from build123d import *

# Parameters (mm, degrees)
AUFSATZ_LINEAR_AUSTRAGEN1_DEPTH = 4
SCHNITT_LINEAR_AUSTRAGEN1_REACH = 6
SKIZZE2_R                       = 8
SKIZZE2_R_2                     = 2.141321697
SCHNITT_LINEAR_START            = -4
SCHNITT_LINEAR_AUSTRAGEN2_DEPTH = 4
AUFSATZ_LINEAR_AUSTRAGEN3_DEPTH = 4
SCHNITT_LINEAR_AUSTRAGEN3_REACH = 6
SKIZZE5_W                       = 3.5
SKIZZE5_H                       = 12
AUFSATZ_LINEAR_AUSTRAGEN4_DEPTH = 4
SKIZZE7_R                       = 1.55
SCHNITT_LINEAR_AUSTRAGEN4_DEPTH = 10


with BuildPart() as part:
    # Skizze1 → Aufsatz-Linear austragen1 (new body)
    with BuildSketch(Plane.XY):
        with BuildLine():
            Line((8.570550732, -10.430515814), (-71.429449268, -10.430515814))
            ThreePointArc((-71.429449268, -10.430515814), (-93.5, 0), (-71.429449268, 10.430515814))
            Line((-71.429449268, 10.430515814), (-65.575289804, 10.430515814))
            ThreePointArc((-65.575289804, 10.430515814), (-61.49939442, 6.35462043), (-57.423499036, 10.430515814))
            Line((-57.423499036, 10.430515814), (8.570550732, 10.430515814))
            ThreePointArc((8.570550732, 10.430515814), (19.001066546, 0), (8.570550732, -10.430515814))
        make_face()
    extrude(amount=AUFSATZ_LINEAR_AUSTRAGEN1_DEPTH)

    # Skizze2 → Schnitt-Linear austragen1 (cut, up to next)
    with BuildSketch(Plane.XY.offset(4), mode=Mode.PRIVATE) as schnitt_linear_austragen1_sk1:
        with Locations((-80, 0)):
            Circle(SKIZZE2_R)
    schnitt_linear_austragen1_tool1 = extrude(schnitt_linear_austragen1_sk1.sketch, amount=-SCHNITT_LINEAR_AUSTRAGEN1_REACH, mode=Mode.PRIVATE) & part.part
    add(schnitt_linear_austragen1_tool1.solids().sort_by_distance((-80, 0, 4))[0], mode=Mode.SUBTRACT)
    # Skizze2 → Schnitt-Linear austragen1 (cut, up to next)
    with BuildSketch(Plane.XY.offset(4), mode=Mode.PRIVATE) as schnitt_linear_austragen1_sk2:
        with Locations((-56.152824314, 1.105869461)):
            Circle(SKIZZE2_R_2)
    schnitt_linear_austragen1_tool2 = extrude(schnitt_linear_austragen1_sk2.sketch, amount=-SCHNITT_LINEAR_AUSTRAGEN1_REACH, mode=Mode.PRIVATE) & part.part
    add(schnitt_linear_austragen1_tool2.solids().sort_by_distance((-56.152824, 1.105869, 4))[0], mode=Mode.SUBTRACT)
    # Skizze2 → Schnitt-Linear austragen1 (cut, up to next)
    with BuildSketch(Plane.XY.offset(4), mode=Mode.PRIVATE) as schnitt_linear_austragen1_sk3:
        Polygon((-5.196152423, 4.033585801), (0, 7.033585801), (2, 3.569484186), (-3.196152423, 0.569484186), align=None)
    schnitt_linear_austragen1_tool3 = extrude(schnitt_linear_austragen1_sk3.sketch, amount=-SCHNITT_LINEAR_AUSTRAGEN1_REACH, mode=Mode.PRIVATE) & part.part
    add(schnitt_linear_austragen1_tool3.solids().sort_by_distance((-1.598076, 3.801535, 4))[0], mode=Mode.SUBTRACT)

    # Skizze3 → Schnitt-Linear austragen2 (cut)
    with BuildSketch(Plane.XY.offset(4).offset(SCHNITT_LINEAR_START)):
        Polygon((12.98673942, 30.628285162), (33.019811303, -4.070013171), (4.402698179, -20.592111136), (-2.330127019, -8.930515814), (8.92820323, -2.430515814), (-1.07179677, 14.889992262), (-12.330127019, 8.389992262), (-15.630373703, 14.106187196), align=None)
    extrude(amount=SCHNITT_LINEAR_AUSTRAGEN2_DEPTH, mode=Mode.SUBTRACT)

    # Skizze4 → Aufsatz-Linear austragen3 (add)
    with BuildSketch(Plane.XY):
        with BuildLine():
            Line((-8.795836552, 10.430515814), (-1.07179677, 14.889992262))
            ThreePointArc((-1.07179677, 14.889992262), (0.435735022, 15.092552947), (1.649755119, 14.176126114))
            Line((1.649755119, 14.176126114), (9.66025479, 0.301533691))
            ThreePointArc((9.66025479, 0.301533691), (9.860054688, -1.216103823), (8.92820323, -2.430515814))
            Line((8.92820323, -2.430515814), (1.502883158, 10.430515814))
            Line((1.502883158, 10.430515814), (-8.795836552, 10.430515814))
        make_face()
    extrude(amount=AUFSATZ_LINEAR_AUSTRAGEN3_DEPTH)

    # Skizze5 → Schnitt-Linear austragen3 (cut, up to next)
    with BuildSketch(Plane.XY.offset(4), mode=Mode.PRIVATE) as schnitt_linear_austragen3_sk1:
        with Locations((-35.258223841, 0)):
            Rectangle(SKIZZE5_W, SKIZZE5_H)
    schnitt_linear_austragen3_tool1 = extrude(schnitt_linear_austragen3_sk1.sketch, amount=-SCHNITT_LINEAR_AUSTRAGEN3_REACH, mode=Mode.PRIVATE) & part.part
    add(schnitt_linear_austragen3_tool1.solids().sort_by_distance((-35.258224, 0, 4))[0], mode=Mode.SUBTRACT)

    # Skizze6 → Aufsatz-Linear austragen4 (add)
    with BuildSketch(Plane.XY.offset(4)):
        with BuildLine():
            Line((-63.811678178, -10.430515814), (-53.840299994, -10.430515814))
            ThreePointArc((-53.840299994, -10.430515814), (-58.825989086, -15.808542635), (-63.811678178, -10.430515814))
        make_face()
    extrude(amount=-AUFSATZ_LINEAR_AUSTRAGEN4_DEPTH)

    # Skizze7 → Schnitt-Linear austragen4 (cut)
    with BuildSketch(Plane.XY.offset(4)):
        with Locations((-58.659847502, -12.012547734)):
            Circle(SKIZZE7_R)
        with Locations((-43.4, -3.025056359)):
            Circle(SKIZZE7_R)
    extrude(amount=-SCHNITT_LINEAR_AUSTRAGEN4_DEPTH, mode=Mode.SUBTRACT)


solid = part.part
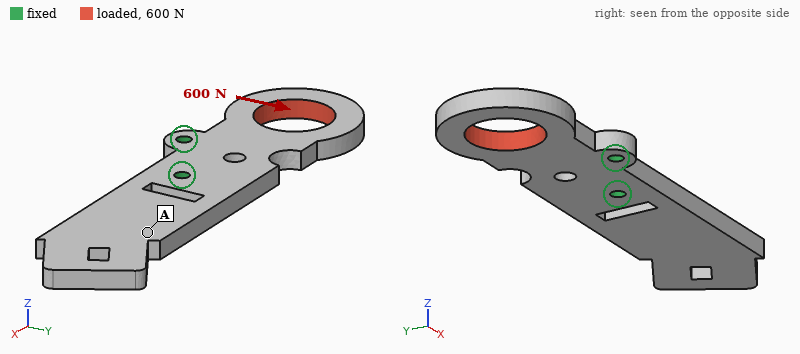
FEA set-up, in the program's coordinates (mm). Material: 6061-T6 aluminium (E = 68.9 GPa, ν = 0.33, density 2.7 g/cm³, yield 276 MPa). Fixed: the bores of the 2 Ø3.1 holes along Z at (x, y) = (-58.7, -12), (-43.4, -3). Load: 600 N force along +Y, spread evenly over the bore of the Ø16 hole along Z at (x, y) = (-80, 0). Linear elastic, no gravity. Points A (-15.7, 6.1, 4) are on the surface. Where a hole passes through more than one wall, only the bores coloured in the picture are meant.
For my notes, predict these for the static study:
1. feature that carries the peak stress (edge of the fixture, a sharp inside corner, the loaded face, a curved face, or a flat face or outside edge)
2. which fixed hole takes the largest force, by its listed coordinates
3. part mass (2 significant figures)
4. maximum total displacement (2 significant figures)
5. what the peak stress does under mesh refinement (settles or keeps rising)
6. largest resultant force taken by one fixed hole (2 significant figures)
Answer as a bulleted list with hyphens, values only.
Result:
- a sharp inside corner
- (-58.7, -12)
- 20 g
- 85 µm
- keeps rising
- 1.2 kN
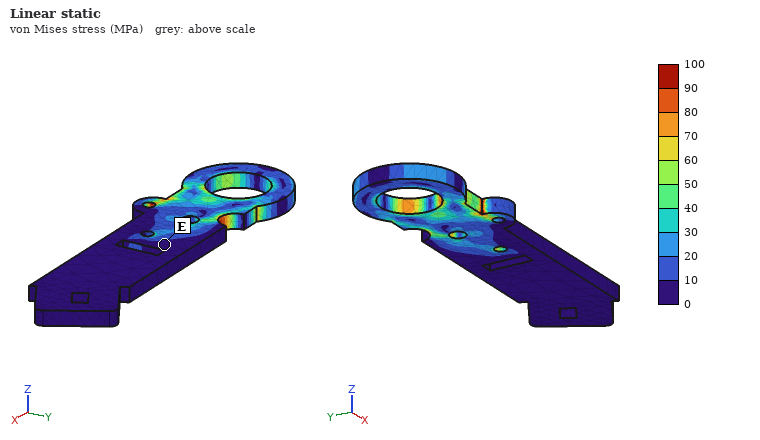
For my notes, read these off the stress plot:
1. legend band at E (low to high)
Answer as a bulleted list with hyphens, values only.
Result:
- 0 to 10 MPa
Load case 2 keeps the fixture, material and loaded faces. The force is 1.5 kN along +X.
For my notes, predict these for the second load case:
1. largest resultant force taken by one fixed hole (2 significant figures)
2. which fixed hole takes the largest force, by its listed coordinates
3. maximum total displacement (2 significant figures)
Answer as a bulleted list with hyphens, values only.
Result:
- 1.2 kN
- (-43.4, -3)
- 44 µm
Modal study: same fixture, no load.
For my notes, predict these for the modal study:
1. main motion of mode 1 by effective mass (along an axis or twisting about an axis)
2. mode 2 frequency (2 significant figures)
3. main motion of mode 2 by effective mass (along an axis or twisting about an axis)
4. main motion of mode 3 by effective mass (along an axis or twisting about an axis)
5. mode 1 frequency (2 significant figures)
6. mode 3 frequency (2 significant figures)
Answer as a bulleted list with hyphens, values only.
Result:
- along Z
- 2300 Hz
- along Z
- along Y
- 1000 Hz
- 4100 Hz
